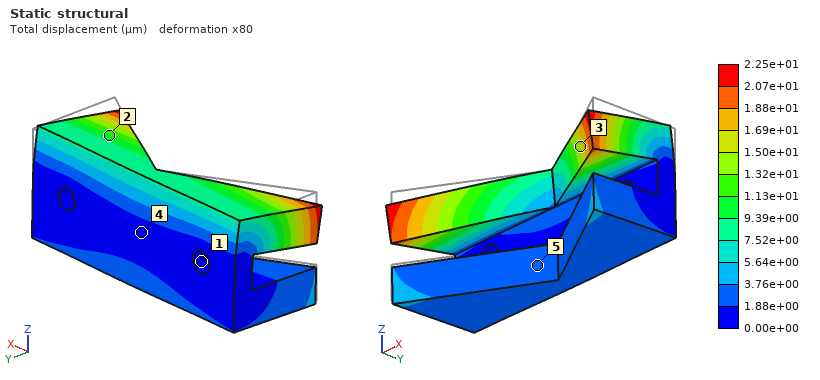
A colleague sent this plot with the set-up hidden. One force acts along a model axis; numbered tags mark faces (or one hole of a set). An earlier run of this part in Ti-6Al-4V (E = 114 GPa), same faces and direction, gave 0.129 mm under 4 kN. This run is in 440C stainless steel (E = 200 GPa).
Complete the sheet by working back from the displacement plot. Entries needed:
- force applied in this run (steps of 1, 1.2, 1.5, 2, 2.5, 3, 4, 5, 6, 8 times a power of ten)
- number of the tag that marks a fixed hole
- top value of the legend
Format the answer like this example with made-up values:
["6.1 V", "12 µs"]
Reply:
["1.2 kN", "1", "2.25e+01 µm"]
